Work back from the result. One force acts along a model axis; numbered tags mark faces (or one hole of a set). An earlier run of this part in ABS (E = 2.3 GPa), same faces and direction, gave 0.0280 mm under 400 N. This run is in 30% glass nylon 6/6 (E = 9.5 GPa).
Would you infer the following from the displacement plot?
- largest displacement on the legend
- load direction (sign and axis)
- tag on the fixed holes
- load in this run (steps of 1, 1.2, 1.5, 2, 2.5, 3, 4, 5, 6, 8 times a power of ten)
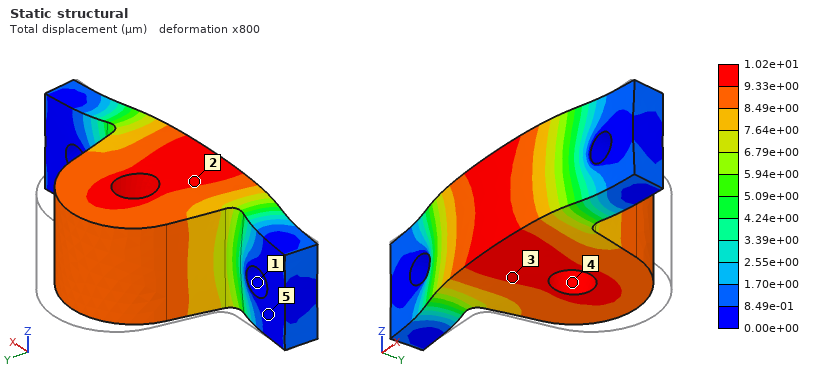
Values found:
1.02e+01 µm
-Y
1
600 N
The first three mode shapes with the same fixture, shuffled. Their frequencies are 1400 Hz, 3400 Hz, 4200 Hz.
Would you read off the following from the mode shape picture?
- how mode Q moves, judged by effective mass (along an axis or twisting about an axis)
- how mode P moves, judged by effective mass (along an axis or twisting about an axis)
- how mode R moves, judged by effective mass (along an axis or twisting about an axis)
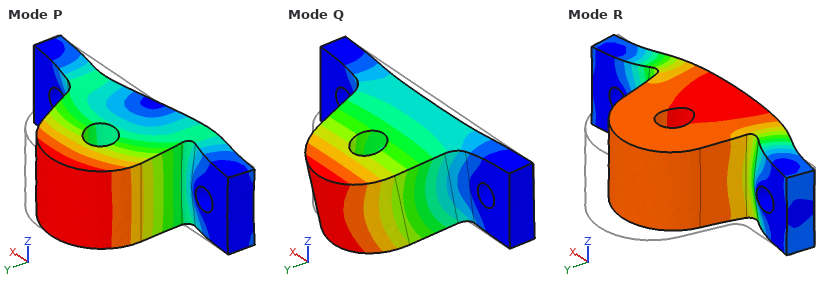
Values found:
along Z
along X
along Y
